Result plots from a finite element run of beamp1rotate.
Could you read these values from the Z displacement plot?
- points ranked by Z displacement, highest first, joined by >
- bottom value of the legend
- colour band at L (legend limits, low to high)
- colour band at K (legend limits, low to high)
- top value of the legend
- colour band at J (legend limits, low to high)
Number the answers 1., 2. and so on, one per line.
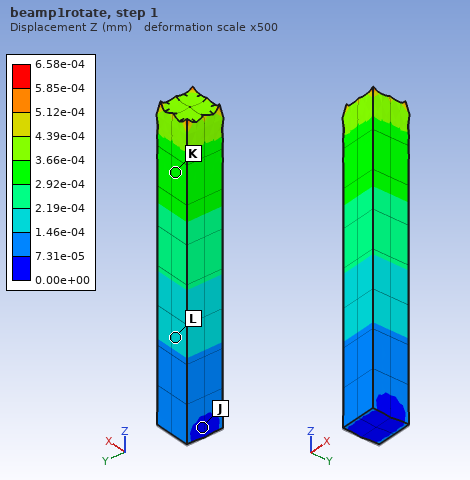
1. K > L > J
2. 0.00e+00 mm
3. 1.46e-04 to 2.19e-04 mm
4. 2.92e-04 to 3.66e-04 mm
5. 6.58e-04 mm
6. 0.00e+00 to 7.31e-05 mm
